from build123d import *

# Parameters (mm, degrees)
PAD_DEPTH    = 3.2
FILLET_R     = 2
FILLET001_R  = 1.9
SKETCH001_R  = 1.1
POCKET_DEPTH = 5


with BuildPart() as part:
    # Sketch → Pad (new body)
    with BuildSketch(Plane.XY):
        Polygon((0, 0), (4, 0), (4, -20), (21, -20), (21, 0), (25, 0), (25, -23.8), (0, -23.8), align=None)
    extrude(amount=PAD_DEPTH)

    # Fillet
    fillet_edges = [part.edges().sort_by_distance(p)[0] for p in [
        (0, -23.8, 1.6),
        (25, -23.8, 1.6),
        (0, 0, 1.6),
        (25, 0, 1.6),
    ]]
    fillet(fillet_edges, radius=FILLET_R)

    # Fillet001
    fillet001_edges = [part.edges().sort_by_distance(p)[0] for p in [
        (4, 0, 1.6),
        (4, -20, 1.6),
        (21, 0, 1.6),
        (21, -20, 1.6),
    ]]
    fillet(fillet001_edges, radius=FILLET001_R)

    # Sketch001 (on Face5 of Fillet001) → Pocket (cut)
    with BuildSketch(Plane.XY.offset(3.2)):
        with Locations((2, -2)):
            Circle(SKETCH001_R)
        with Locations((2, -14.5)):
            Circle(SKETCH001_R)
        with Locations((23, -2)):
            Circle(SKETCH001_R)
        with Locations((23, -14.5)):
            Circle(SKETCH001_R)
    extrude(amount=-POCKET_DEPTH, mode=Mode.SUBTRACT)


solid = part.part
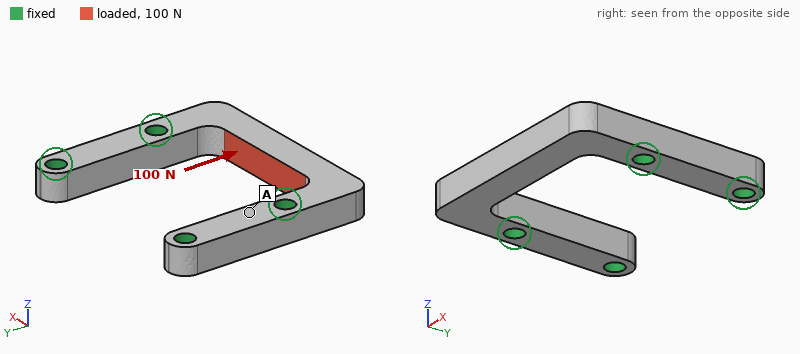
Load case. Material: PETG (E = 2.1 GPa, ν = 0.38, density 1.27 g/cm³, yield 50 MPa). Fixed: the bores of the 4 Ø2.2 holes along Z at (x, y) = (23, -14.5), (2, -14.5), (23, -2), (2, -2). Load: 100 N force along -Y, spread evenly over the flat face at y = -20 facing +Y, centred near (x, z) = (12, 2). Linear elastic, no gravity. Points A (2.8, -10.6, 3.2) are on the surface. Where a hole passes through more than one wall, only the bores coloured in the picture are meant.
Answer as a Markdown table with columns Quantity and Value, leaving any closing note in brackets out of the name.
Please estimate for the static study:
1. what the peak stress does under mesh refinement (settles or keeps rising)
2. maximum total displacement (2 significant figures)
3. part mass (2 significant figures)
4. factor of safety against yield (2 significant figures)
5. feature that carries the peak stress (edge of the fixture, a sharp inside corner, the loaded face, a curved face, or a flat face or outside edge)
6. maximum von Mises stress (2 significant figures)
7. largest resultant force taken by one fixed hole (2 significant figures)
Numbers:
| Quantity | Value |
|---|---|
| what the peak stress does under mesh refinement | settles |
| maximum total displacement | 0.15 mm |
| part mass | 0.96 g |
| factor of safety against yield | 1.7 |
| feature that carries the peak stress | a curved face |
| maximum von Mises stress | 29 MPa |
| largest resultant force taken by one fixed hole | 62 N |
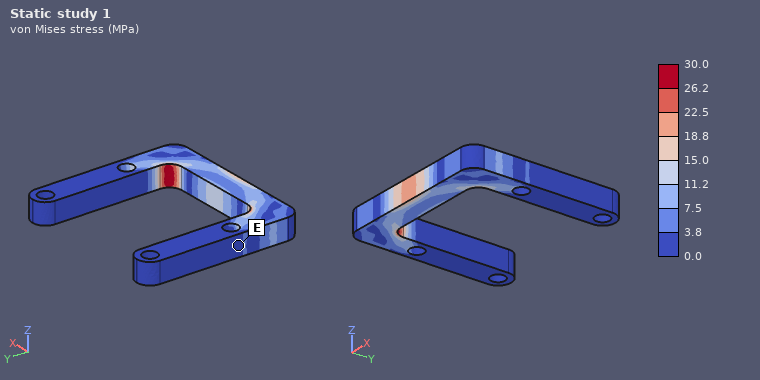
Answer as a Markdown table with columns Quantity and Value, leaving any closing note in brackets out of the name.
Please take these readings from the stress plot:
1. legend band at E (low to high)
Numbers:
| Quantity | Value |
|---|---|
| legend band at E | 0.0 to 3.8 MPa |
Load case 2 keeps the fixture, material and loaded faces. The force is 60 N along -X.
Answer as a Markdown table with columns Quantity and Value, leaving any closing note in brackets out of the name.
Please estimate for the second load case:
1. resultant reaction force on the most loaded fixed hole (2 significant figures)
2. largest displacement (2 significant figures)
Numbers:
| Quantity | Value |
|---|---|
| resultant reaction force on the most loaded fixed hole | 31 N |
| largest displacement | 81 µm |
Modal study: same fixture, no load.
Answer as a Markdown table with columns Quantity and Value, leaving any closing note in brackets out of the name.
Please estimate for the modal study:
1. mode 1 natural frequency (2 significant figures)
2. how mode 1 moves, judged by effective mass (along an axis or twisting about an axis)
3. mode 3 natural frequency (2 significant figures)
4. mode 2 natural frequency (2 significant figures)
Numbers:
| Quantity | Value |
|---|---|
| mode 1 natural frequency | 4100 Hz |
| how mode 1 moves, judged by effective mass | along Z |
| mode 3 natural frequency | 7800 Hz |
| mode 2 natural frequency | 7600 Hz |
